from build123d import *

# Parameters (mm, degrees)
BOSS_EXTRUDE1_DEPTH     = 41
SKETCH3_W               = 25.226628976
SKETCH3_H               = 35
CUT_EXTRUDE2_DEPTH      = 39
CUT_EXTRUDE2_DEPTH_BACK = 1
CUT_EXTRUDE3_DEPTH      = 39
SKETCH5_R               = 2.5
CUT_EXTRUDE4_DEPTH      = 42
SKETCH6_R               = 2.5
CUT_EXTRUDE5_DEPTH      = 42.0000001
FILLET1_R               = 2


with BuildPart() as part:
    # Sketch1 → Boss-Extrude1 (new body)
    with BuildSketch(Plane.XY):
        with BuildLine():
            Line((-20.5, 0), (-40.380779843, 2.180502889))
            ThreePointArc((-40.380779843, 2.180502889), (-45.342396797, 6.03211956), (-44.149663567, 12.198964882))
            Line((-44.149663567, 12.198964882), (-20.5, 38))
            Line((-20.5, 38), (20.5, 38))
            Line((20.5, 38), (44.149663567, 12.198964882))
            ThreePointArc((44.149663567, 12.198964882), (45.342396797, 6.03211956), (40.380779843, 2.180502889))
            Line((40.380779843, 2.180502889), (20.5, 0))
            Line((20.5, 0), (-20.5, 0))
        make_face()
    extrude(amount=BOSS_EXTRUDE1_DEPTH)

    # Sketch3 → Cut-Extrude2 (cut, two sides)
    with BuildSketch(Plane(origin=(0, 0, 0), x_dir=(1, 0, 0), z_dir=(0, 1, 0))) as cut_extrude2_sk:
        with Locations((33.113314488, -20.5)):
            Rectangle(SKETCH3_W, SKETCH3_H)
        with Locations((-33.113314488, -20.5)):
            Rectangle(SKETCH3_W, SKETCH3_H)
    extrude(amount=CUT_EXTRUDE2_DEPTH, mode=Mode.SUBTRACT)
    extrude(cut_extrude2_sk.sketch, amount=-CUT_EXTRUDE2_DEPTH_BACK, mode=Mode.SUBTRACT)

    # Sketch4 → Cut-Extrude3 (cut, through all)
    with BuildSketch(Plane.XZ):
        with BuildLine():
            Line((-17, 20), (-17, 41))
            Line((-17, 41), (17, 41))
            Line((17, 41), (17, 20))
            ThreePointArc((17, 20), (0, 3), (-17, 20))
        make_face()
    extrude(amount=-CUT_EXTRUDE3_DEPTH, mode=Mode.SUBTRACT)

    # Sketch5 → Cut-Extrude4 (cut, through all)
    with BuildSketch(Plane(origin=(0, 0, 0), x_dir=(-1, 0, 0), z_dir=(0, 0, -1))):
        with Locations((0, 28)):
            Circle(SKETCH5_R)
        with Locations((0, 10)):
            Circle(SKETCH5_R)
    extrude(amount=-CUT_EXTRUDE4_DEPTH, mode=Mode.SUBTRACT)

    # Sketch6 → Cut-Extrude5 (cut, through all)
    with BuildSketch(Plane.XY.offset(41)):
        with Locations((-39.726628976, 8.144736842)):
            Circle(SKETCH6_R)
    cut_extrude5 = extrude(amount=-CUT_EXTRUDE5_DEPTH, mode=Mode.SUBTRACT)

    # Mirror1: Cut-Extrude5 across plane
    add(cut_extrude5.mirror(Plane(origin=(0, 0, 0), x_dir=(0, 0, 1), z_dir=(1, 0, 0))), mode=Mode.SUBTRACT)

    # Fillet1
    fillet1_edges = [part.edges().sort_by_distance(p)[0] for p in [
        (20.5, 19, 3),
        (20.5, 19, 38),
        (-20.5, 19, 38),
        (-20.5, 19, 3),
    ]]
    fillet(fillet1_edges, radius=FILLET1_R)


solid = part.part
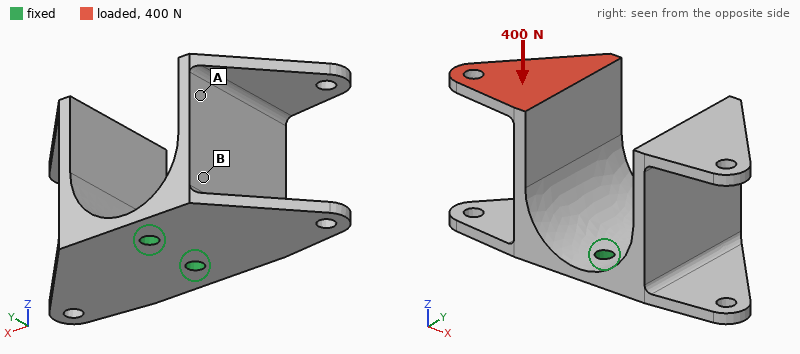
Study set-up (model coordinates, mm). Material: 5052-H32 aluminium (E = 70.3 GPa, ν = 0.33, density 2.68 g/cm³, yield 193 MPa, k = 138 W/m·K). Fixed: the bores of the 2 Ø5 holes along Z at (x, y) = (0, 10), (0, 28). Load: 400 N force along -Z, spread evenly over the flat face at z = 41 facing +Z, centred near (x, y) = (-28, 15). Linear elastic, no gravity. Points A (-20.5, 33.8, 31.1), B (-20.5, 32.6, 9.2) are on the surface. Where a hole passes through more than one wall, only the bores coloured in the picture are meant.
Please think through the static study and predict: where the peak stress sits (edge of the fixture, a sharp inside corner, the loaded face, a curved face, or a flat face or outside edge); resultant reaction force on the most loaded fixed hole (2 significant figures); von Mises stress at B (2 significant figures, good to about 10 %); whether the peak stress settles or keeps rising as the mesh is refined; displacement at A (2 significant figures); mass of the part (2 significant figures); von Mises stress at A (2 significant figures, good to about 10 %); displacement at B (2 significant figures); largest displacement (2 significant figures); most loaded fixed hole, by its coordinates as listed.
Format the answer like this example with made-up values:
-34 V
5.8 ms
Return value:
edge of the fixture
260 N
17 MPa
keeps rising
0.29 mm
70 g
38 MPa
0.13 mm
0.79 mm
(0, 10)
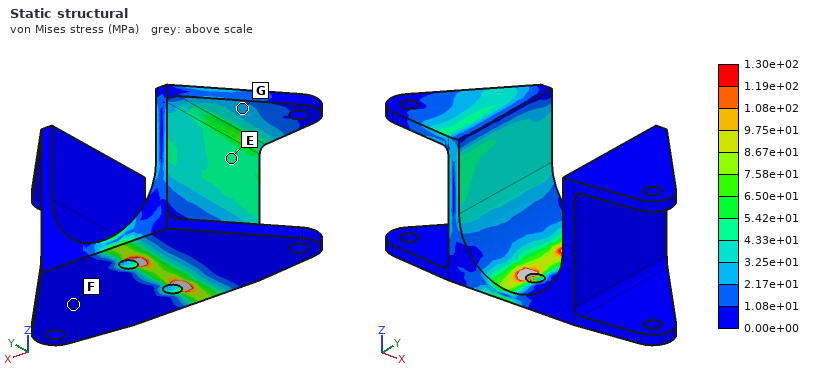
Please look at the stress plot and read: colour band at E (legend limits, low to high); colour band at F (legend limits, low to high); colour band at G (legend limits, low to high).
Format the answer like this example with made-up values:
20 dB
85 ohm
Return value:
4.33e+01 to 5.42e+01 MPa
0.00e+00 to 1.08e+01 MPa
2.17e+01 to 3.25e+01 MPa
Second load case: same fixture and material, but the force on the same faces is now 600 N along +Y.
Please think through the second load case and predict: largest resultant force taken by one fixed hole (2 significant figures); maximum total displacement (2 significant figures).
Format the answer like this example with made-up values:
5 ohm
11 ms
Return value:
1.4 kN
0.24 mm
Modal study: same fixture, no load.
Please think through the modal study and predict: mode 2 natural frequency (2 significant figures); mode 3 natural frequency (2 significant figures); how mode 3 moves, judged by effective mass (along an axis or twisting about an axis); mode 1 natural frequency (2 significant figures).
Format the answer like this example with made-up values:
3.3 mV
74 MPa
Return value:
1100 Hz
3100 Hz
twisting about Z
1000 Hz
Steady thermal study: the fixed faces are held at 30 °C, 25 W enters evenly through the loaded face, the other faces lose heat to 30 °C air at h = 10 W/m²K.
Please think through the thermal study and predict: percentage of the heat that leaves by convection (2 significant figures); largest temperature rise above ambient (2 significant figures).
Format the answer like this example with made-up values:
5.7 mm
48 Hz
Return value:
7.6 %
74 K
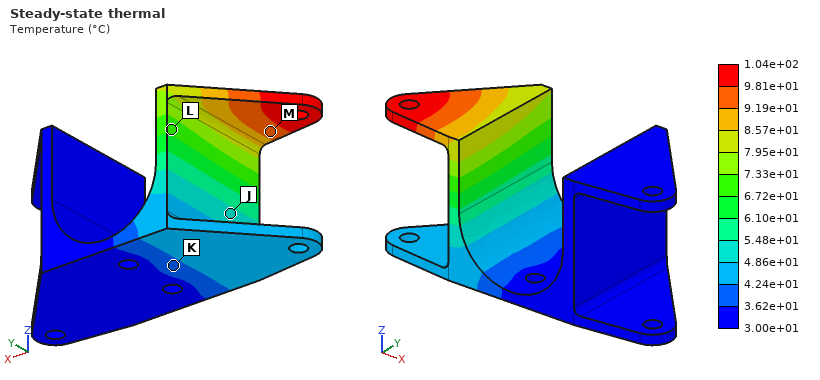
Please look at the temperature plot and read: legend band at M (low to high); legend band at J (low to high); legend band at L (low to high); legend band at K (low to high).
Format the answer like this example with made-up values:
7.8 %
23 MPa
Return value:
9.19e+01 to 9.81e+01 °C
4.86e+01 to 5.48e+01 °C
6.72e+01 to 7.33e+01 °C
3.62e+01 to 4.24e+01 °C
